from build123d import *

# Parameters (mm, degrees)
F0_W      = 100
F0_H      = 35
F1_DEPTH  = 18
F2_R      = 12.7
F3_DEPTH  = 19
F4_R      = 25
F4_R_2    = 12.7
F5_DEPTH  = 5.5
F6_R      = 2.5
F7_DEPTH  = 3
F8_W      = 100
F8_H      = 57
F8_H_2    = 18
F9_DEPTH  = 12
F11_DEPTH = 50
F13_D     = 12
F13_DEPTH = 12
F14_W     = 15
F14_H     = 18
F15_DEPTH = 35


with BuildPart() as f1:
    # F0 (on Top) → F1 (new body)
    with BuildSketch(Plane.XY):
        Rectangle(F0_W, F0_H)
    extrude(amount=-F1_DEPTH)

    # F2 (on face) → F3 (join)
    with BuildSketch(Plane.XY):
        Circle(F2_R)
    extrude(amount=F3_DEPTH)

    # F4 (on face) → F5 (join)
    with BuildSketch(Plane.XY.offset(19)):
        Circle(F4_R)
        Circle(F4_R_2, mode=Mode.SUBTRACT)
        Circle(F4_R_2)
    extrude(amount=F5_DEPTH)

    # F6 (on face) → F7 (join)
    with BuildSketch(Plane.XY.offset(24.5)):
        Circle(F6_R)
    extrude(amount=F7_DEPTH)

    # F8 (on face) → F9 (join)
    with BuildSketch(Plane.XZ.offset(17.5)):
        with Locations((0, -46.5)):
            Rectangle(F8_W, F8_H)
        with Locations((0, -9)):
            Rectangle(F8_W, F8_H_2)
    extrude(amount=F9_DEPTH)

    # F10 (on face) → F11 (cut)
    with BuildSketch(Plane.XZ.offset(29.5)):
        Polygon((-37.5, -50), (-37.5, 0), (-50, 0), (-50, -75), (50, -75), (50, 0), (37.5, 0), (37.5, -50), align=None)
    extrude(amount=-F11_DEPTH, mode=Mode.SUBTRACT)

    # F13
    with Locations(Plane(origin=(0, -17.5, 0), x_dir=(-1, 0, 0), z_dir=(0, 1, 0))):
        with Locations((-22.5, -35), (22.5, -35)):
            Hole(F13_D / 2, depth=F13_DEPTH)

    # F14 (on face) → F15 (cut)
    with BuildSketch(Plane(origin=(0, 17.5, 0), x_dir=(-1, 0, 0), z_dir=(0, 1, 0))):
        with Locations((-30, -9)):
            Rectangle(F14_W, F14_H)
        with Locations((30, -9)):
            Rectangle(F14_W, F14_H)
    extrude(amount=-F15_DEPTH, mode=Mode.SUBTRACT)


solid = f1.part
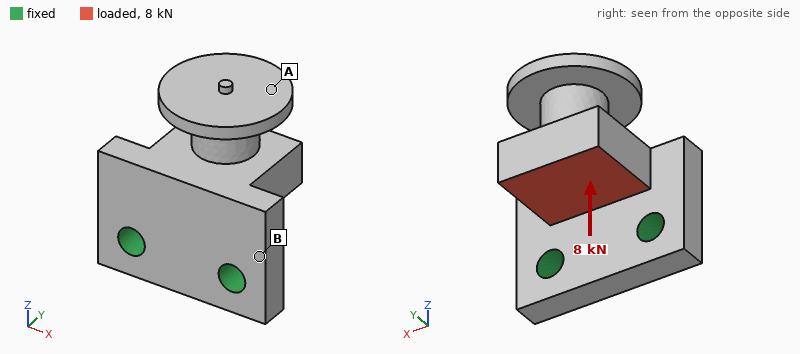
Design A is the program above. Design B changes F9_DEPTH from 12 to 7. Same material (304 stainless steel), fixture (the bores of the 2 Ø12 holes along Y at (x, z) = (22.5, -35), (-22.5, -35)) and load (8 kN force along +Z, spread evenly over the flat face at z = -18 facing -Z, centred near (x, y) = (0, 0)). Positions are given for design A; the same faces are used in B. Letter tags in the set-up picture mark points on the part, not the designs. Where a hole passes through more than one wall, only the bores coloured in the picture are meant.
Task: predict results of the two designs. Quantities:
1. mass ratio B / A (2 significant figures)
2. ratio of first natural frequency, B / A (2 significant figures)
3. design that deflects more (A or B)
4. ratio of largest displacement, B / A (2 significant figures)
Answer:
0.81
0.54
B
3.3
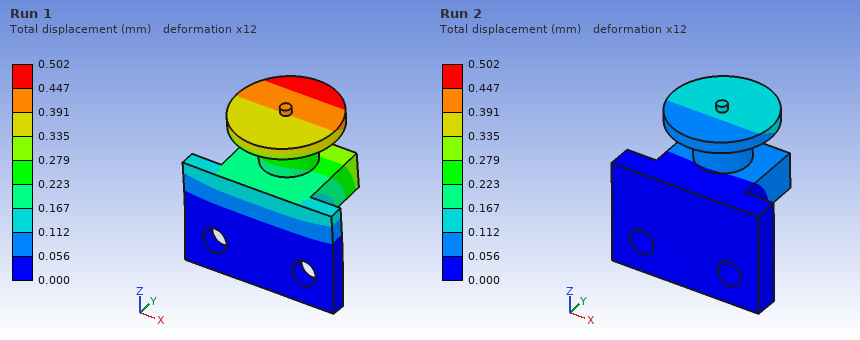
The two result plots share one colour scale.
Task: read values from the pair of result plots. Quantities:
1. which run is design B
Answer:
Run 1
